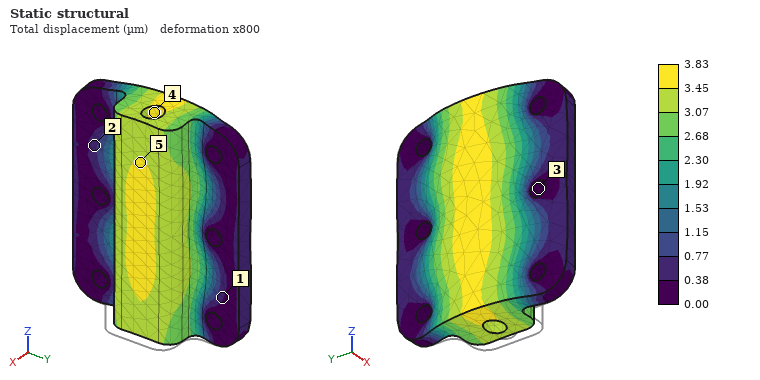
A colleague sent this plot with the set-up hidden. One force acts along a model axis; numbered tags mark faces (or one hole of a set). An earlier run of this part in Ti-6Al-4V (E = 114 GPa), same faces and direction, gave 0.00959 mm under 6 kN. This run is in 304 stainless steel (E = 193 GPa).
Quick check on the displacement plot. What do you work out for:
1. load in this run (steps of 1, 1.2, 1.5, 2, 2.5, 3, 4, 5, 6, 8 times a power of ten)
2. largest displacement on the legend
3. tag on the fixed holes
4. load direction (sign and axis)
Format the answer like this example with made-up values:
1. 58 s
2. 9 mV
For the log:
1. 4 kN
2. 3.83 µm
3. 3
4. -X
